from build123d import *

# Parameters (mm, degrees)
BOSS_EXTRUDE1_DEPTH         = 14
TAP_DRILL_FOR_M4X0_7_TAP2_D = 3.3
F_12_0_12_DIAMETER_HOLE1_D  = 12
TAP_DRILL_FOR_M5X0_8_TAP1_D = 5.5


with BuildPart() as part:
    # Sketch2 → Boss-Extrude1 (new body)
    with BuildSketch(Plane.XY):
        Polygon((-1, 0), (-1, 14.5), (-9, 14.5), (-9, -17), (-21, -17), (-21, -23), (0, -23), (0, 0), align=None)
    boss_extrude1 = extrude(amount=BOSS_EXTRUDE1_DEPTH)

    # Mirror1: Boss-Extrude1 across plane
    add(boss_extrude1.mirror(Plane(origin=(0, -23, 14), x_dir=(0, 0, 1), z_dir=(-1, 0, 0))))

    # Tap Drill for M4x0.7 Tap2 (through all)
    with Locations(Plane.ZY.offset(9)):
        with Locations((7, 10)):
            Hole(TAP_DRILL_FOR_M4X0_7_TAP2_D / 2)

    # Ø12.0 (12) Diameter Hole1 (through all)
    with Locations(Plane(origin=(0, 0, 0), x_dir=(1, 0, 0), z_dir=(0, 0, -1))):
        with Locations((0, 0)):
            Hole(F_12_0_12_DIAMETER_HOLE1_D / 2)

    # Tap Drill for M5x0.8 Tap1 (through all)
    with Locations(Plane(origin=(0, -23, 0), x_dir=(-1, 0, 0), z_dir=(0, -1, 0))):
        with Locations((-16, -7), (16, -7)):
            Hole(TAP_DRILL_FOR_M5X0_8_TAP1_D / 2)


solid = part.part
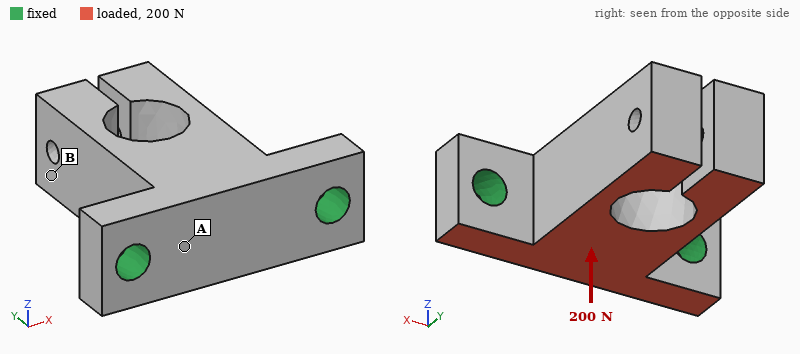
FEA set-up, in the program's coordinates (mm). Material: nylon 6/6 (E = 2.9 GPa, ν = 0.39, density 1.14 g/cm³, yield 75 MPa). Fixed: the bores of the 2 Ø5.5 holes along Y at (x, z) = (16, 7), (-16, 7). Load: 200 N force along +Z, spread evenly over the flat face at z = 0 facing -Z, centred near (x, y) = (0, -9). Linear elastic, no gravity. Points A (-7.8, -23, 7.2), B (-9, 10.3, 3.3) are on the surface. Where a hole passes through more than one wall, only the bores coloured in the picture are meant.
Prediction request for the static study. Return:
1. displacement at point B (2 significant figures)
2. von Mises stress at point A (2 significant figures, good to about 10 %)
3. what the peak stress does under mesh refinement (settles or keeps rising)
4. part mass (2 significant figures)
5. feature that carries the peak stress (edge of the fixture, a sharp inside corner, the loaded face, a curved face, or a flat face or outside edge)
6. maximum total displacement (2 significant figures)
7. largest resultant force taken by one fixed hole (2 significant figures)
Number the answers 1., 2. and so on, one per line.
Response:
1. 0.33 mm
2. 4.4 MPa
3. keeps rising
4. 11 g
5. edge of the fixture
6. 0.40 mm
7. 100 N
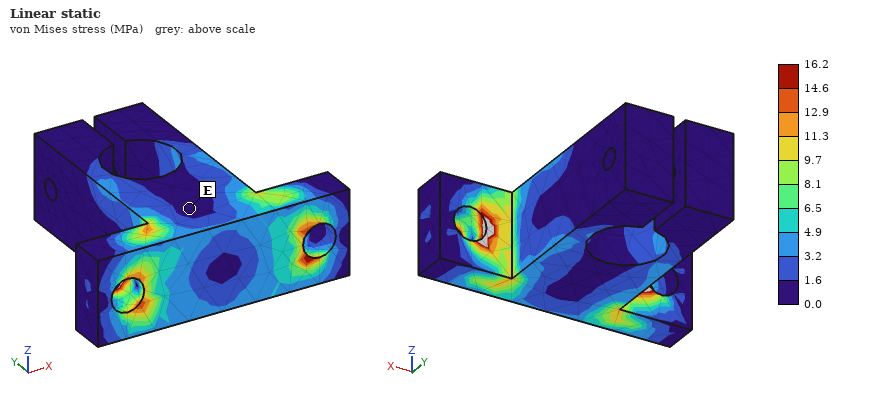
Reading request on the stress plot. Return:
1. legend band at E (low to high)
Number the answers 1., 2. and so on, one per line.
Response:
1. 0.0 to 1.6 MPa
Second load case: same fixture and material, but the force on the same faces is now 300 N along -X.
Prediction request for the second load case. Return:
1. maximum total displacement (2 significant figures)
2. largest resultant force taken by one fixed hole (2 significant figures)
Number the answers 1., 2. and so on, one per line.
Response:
1. 0.66 mm
2. 220 N
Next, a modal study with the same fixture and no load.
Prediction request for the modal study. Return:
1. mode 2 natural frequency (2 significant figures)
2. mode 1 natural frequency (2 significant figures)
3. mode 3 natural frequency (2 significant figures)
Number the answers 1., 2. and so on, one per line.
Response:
1. 1400 Hz
2. 1300 Hz
3. 1500 Hz
